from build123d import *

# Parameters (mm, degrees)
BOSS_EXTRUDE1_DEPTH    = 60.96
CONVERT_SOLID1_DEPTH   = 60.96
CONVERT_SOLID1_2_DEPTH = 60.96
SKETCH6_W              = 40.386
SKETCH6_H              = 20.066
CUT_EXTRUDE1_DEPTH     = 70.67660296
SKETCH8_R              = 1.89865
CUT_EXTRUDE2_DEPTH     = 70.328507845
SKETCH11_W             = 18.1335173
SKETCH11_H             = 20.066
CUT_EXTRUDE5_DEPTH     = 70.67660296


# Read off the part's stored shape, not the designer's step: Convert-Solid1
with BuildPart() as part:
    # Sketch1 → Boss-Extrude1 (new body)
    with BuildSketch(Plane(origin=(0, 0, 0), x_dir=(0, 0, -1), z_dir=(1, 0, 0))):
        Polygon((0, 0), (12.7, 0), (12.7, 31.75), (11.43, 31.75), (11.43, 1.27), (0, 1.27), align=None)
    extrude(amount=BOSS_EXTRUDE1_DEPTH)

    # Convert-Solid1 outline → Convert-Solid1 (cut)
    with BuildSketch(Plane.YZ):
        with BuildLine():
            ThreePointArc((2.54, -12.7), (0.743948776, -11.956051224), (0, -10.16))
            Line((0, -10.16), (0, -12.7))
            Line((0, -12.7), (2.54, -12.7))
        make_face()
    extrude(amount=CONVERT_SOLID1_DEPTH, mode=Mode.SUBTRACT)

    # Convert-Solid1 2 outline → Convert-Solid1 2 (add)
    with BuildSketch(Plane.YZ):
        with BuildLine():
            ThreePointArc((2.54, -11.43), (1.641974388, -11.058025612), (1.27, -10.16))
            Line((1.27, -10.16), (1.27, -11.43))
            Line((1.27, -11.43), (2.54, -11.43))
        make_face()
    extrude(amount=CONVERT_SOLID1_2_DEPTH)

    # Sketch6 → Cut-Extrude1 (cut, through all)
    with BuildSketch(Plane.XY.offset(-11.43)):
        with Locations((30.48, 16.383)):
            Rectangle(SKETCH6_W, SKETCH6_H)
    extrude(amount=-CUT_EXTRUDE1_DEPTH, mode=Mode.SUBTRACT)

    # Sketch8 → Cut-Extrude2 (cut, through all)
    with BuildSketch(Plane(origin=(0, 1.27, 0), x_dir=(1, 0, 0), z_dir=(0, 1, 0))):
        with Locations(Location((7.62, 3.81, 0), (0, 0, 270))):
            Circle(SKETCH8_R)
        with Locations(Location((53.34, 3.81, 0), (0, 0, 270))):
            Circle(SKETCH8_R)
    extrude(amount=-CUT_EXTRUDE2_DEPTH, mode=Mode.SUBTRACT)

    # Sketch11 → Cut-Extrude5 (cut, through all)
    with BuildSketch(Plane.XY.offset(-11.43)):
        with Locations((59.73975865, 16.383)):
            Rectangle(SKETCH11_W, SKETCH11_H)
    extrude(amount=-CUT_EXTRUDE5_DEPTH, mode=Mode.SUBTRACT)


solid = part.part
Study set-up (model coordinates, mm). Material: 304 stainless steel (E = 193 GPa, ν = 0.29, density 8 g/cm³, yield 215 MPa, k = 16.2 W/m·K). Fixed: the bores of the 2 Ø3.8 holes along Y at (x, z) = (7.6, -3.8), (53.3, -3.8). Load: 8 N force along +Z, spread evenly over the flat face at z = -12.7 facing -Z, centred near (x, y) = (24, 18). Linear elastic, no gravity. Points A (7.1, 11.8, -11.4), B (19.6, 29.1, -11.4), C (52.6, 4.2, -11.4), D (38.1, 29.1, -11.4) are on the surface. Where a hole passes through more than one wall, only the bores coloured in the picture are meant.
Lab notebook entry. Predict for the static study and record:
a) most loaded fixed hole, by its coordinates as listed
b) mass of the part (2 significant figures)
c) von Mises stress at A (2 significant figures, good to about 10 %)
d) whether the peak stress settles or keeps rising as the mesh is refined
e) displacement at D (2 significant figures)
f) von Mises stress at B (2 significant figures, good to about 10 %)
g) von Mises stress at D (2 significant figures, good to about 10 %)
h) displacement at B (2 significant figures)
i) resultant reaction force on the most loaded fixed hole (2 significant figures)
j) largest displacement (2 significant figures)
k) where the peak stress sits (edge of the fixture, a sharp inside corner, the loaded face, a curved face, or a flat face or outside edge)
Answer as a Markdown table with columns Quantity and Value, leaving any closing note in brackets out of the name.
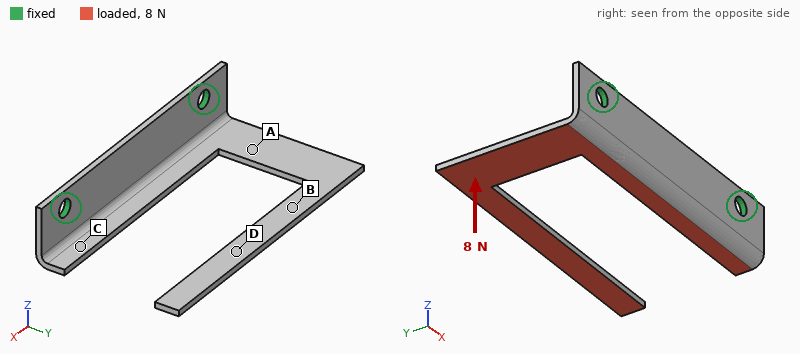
| Quantity | Value |
|---|---|
| most loaded fixed hole, by its coordinates as listed | (7.6, -3.8) |
| mass of the part | 16 g |
| von Mises stress at A | 40 MPa |
| whether the peak stress settles or keeps rising as the mesh is refined | keeps rising |
| displacement at D | 0.38 mm |
| von Mises stress at B | 33 MPa |
| von Mises stress at D | 10 MPa |
| displacement at B | 0.20 mm |
| resultant reaction force on the most loaded fixed hole | 6.4 N |
| largest displacement | 0.67 mm |
| where the peak stress sits | a sharp inside corner |
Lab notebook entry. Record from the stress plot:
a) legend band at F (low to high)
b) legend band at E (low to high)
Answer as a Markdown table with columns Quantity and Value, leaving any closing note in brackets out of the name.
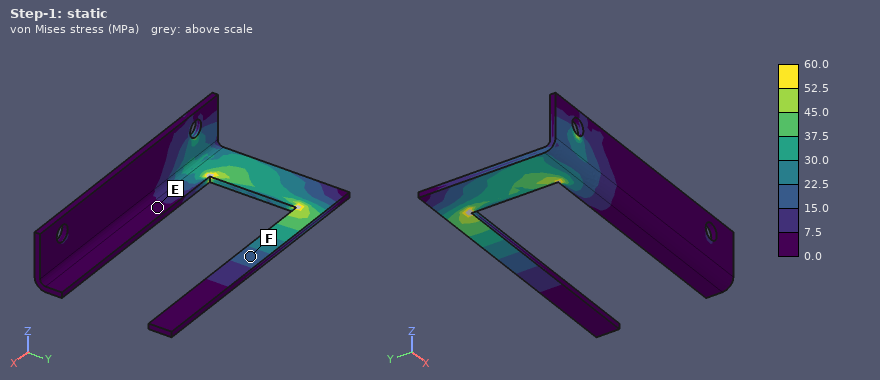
| Quantity | Value |
|---|---|
| legend band at F | 15.0 to 22.5 MPa |
| legend band at E | 0.0 to 7.5 MPa |
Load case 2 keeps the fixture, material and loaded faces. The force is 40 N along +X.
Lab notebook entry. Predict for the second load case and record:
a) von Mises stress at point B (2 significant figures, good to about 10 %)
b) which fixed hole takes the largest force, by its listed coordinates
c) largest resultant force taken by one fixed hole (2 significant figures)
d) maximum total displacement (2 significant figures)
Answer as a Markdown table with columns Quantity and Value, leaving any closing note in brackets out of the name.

| Quantity | Value |
|---|---|
| von Mises stress at point B | 3.4 MPa |
| which fixed hole takes the largest force, by its listed coordinates | (53.3, -3.8) |
| largest resultant force taken by one fixed hole | 48 N |
| maximum total displacement | 0.11 mm |
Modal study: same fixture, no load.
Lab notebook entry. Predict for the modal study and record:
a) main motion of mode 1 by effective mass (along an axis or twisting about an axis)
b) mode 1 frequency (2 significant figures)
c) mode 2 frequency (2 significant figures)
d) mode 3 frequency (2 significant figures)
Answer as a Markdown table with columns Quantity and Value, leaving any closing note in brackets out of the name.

| Quantity | Value |
|---|---|
| main motion of mode 1 by effective mass | along Z |
| mode 1 frequency | 250 Hz |
| mode 2 frequency | 720 Hz |
| mode 3 frequency | 1100 Hz |
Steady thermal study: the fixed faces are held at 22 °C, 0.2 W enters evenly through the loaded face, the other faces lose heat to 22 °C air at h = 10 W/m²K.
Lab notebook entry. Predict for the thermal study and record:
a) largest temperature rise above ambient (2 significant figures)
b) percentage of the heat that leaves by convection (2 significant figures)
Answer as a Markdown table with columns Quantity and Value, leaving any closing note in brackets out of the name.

| Quantity | Value |
|---|---|
| largest temperature rise above ambient | 13 K |
| percentage of the heat that leaves by convection | 45 % |
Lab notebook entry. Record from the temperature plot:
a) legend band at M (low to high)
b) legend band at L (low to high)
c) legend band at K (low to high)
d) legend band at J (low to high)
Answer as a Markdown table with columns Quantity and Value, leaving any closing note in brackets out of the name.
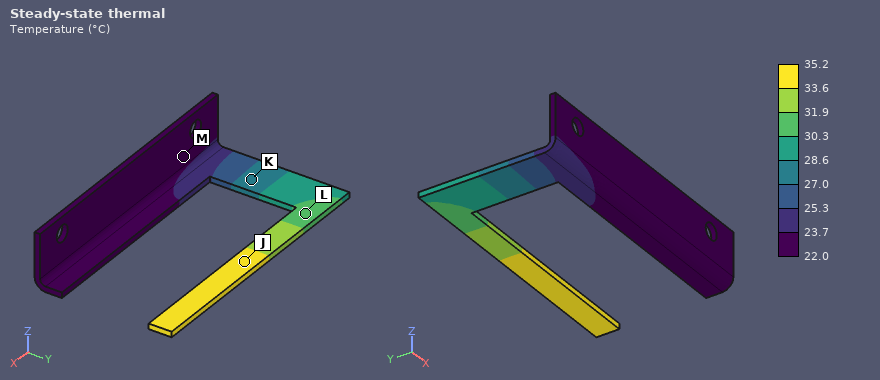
| Quantity | Value |
|---|---|
| legend band at M | 22.0 to 23.7 °C |
| legend band at L | 30.3 to 31.9 °C |
| legend band at K | 27.0 to 28.6 °C |
| legend band at J | 33.6 to 35.2 °C |
